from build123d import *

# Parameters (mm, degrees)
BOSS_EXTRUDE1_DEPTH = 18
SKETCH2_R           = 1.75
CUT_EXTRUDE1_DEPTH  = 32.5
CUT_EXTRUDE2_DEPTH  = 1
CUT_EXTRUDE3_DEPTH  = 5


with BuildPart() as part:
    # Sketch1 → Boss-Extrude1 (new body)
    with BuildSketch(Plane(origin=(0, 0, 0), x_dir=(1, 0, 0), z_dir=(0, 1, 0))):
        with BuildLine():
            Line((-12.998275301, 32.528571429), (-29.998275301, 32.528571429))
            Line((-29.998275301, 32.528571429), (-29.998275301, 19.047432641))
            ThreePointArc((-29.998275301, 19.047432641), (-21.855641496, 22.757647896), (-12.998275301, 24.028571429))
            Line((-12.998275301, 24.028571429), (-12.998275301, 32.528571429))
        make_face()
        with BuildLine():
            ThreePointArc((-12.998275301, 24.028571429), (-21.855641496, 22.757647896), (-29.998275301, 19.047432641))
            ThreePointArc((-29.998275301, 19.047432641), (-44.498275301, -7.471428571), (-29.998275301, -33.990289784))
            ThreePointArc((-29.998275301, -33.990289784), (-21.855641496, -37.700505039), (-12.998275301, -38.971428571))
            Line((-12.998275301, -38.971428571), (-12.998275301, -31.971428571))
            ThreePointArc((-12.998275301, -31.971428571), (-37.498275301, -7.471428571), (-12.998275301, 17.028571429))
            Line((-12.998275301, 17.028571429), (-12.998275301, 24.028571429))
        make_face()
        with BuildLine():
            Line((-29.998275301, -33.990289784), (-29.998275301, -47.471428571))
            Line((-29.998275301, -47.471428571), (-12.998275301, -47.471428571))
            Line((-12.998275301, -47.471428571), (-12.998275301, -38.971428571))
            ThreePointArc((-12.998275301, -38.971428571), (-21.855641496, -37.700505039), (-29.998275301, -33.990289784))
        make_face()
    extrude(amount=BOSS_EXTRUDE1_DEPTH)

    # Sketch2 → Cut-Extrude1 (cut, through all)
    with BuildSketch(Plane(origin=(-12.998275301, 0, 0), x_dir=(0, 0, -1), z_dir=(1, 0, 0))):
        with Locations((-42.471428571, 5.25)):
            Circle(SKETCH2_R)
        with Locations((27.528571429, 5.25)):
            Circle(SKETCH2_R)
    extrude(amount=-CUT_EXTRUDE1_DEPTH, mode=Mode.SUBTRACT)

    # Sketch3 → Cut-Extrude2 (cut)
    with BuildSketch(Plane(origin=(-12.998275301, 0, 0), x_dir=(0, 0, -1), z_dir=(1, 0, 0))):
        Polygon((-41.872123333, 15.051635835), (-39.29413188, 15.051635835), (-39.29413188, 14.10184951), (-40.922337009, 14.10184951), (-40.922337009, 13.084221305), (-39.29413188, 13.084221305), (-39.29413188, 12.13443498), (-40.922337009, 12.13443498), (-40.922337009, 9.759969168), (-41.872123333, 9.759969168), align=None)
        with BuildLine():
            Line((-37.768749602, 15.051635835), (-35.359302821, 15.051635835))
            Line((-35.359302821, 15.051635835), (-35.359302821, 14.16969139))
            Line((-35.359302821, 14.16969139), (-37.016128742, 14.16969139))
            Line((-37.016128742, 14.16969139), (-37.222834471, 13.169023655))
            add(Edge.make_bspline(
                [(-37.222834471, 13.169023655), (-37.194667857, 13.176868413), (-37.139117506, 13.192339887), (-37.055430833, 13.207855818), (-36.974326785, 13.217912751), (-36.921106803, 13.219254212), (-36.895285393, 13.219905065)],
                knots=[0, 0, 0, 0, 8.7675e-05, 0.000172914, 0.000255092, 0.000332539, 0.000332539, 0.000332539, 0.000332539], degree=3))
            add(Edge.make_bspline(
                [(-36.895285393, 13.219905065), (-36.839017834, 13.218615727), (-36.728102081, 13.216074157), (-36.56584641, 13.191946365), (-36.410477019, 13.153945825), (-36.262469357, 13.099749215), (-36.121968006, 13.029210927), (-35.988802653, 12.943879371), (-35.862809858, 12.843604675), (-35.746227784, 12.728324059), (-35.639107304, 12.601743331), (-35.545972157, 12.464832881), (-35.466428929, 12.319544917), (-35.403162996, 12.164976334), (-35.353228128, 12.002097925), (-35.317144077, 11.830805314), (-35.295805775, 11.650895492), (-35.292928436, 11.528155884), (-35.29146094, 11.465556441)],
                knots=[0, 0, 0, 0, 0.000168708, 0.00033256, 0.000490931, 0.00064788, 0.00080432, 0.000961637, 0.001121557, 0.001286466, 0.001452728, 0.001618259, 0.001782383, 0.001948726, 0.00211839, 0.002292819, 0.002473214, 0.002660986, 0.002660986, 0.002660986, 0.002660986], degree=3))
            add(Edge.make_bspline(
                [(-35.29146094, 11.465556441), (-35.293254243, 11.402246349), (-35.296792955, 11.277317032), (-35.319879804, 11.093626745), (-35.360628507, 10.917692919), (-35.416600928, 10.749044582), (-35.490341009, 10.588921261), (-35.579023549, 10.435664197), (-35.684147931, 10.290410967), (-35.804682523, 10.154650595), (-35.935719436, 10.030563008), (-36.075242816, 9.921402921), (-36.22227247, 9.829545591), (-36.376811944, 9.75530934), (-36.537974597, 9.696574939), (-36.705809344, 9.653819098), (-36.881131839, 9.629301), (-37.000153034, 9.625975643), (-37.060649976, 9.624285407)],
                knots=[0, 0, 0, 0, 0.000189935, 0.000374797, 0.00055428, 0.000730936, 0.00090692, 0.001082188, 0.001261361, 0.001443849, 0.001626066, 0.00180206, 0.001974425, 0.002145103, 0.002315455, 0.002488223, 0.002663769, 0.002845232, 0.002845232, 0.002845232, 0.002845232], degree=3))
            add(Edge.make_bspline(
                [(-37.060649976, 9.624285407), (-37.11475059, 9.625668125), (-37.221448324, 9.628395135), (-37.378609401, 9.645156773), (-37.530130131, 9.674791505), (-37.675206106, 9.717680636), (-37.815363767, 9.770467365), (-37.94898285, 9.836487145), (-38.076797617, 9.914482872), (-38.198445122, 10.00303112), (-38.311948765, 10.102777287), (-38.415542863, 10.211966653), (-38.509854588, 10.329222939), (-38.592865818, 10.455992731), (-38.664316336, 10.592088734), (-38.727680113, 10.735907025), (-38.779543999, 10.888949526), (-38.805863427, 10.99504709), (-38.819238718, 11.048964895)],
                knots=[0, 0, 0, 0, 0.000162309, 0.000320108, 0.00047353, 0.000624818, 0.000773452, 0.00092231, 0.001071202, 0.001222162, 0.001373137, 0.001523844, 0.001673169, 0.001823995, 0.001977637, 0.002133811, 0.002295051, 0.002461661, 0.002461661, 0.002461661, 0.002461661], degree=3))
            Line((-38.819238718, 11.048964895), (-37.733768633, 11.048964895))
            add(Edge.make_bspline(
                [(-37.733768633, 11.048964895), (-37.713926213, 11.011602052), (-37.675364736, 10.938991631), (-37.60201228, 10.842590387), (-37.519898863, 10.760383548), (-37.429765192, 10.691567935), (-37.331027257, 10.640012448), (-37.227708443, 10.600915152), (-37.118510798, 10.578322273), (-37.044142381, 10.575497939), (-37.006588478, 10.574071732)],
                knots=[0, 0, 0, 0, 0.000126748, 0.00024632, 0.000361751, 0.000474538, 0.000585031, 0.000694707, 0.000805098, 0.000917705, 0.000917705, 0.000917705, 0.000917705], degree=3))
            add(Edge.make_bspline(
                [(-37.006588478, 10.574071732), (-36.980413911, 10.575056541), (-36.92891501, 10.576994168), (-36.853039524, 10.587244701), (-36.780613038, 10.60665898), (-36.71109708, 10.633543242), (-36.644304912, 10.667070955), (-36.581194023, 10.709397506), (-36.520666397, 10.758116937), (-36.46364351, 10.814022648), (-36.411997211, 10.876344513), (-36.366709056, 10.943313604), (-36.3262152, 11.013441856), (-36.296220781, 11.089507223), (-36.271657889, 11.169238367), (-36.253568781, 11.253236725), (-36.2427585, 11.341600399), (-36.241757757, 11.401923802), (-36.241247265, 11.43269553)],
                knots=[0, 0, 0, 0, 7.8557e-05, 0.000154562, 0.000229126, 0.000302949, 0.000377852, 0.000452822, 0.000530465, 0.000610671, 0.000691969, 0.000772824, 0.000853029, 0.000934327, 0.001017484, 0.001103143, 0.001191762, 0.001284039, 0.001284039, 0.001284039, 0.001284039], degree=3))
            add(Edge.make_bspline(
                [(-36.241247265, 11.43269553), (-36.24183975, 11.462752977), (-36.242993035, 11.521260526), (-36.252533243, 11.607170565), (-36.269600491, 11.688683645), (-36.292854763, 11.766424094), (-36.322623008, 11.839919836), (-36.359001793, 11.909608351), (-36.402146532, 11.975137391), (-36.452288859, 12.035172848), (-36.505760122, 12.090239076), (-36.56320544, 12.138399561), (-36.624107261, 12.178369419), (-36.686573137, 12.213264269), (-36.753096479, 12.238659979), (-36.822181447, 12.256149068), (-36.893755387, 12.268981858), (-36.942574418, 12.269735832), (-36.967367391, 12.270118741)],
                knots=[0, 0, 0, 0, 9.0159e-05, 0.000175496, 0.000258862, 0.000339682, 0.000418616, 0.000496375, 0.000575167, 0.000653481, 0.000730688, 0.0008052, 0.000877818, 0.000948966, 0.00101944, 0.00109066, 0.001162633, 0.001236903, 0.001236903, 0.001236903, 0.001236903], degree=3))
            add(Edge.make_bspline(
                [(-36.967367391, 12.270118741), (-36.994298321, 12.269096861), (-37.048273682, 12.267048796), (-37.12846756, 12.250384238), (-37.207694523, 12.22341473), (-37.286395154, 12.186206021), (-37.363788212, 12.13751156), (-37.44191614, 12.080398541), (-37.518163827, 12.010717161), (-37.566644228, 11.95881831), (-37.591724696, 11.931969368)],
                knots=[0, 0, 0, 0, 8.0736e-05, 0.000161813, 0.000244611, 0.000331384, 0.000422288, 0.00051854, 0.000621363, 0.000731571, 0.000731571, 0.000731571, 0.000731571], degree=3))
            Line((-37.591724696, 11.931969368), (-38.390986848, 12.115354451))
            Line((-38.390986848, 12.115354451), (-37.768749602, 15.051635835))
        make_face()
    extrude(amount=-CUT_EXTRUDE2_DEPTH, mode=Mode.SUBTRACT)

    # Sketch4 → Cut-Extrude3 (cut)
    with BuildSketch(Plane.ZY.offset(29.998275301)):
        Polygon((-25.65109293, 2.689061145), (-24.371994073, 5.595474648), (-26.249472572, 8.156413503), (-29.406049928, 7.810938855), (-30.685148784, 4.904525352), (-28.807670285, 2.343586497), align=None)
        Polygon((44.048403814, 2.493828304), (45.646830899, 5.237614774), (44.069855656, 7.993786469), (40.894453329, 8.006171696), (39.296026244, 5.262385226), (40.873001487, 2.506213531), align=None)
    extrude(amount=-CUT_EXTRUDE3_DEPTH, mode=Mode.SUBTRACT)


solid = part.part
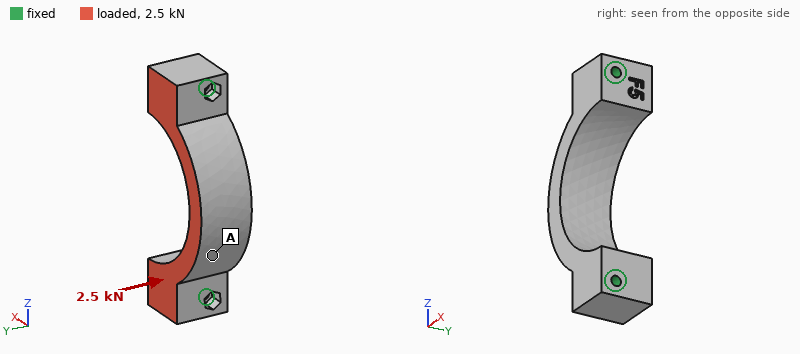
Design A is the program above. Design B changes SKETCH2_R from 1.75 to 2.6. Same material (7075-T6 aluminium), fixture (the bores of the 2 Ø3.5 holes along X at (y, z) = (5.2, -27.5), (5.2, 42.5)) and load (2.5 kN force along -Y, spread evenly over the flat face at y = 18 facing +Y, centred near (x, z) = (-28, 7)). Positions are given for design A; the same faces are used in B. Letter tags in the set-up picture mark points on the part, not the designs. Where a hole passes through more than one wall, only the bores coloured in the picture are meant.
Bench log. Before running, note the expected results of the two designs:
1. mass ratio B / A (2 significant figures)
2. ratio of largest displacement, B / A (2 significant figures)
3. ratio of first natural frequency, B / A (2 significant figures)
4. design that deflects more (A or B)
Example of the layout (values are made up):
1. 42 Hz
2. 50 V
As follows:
1. 0.98
2. 0.73
3. 1.2
4. A
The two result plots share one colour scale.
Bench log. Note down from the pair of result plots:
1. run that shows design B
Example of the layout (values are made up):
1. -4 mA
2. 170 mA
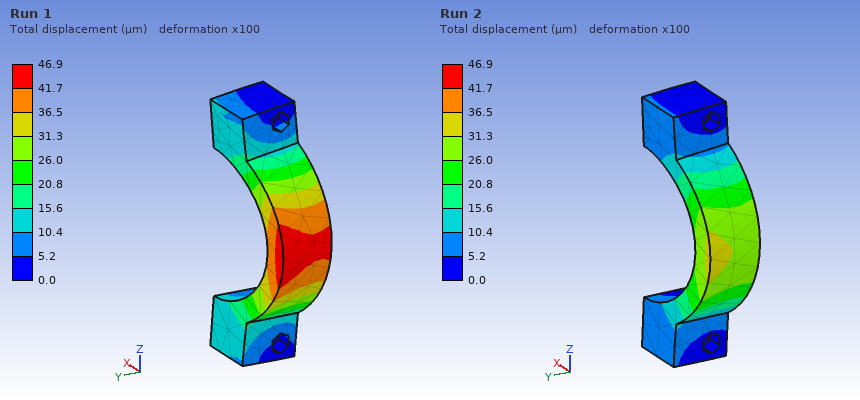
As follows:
1. Run 2
